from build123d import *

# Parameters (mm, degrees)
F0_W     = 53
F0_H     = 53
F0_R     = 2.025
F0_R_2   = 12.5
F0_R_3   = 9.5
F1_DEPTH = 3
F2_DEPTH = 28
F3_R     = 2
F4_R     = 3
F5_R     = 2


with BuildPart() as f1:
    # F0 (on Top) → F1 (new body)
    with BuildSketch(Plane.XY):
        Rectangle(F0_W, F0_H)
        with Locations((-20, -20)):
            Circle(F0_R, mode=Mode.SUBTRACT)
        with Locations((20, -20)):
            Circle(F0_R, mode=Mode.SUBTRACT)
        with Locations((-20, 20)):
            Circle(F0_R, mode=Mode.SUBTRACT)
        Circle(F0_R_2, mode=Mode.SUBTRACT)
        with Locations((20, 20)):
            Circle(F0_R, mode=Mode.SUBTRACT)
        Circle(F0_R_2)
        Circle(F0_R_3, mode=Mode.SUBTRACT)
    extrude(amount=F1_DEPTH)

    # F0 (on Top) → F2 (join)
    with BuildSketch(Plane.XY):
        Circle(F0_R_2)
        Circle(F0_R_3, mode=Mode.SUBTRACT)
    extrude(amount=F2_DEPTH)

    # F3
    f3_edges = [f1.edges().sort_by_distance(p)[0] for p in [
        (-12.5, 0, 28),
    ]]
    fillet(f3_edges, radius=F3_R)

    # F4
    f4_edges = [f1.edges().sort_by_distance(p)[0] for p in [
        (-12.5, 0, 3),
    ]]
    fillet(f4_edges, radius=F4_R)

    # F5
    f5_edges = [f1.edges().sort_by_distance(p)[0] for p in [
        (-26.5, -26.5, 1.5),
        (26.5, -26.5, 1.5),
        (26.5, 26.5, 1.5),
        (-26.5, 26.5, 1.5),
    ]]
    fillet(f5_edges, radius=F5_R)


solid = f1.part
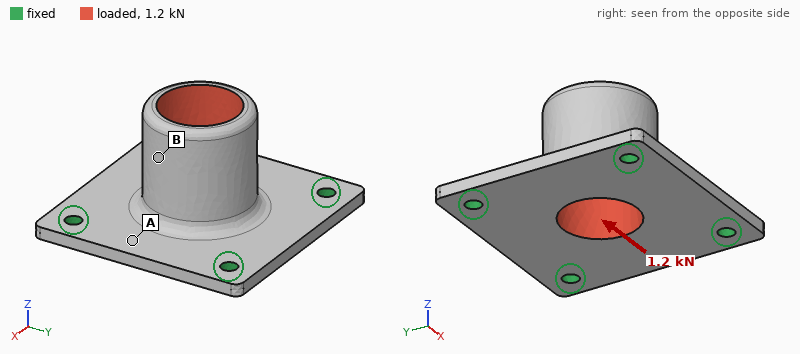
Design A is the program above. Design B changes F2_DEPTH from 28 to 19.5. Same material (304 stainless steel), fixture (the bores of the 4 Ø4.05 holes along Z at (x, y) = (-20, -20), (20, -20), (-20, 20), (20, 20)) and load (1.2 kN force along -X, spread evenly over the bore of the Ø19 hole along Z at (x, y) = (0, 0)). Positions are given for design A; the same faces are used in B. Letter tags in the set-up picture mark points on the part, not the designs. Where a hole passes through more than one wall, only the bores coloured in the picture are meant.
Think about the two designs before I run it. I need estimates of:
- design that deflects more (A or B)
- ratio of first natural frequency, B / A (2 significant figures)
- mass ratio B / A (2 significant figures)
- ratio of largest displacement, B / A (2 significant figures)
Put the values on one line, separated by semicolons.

A; 1.1; 0.86; 0.49
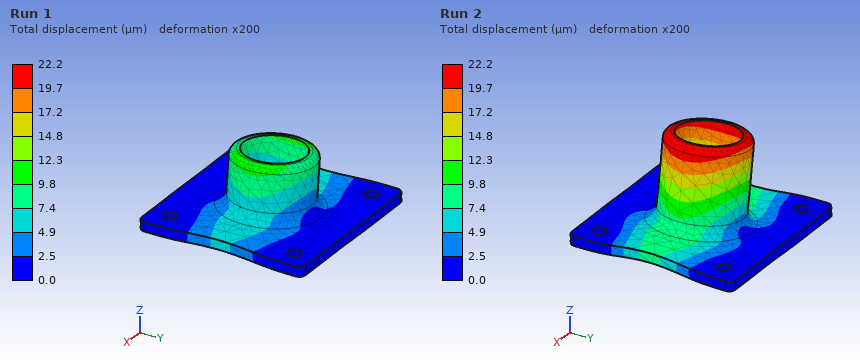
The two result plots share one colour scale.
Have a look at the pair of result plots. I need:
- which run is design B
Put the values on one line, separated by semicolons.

Run 1
